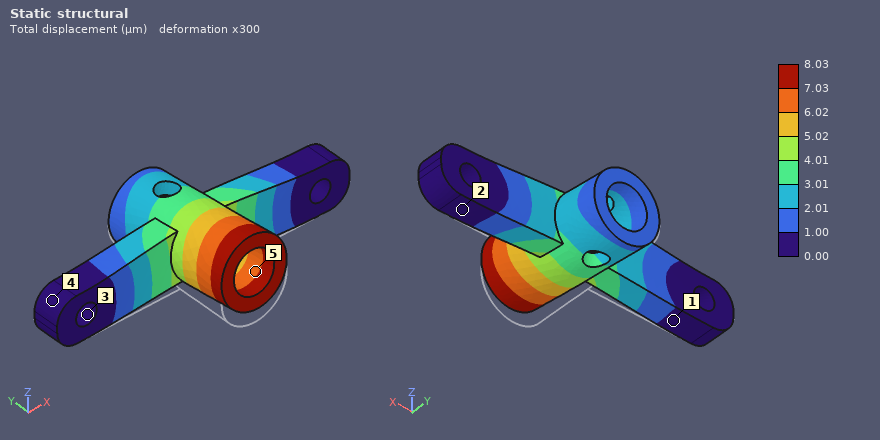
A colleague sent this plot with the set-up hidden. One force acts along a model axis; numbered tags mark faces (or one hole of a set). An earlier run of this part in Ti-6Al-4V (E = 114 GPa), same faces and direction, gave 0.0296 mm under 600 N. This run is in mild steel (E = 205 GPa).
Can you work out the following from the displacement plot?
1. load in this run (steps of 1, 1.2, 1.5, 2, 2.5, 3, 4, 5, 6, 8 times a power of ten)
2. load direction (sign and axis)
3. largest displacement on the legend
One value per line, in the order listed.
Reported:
300 N
+Z
8.03 µm
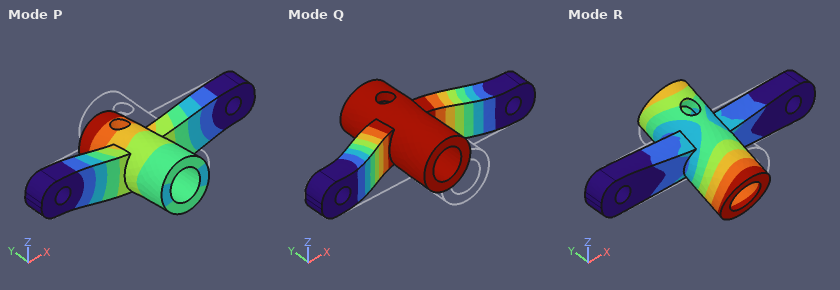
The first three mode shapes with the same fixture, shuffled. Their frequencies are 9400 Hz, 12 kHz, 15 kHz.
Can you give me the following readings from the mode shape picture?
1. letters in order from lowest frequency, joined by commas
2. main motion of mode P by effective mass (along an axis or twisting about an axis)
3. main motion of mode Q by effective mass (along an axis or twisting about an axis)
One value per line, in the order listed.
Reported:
R, Q, P
along Z
along Y
